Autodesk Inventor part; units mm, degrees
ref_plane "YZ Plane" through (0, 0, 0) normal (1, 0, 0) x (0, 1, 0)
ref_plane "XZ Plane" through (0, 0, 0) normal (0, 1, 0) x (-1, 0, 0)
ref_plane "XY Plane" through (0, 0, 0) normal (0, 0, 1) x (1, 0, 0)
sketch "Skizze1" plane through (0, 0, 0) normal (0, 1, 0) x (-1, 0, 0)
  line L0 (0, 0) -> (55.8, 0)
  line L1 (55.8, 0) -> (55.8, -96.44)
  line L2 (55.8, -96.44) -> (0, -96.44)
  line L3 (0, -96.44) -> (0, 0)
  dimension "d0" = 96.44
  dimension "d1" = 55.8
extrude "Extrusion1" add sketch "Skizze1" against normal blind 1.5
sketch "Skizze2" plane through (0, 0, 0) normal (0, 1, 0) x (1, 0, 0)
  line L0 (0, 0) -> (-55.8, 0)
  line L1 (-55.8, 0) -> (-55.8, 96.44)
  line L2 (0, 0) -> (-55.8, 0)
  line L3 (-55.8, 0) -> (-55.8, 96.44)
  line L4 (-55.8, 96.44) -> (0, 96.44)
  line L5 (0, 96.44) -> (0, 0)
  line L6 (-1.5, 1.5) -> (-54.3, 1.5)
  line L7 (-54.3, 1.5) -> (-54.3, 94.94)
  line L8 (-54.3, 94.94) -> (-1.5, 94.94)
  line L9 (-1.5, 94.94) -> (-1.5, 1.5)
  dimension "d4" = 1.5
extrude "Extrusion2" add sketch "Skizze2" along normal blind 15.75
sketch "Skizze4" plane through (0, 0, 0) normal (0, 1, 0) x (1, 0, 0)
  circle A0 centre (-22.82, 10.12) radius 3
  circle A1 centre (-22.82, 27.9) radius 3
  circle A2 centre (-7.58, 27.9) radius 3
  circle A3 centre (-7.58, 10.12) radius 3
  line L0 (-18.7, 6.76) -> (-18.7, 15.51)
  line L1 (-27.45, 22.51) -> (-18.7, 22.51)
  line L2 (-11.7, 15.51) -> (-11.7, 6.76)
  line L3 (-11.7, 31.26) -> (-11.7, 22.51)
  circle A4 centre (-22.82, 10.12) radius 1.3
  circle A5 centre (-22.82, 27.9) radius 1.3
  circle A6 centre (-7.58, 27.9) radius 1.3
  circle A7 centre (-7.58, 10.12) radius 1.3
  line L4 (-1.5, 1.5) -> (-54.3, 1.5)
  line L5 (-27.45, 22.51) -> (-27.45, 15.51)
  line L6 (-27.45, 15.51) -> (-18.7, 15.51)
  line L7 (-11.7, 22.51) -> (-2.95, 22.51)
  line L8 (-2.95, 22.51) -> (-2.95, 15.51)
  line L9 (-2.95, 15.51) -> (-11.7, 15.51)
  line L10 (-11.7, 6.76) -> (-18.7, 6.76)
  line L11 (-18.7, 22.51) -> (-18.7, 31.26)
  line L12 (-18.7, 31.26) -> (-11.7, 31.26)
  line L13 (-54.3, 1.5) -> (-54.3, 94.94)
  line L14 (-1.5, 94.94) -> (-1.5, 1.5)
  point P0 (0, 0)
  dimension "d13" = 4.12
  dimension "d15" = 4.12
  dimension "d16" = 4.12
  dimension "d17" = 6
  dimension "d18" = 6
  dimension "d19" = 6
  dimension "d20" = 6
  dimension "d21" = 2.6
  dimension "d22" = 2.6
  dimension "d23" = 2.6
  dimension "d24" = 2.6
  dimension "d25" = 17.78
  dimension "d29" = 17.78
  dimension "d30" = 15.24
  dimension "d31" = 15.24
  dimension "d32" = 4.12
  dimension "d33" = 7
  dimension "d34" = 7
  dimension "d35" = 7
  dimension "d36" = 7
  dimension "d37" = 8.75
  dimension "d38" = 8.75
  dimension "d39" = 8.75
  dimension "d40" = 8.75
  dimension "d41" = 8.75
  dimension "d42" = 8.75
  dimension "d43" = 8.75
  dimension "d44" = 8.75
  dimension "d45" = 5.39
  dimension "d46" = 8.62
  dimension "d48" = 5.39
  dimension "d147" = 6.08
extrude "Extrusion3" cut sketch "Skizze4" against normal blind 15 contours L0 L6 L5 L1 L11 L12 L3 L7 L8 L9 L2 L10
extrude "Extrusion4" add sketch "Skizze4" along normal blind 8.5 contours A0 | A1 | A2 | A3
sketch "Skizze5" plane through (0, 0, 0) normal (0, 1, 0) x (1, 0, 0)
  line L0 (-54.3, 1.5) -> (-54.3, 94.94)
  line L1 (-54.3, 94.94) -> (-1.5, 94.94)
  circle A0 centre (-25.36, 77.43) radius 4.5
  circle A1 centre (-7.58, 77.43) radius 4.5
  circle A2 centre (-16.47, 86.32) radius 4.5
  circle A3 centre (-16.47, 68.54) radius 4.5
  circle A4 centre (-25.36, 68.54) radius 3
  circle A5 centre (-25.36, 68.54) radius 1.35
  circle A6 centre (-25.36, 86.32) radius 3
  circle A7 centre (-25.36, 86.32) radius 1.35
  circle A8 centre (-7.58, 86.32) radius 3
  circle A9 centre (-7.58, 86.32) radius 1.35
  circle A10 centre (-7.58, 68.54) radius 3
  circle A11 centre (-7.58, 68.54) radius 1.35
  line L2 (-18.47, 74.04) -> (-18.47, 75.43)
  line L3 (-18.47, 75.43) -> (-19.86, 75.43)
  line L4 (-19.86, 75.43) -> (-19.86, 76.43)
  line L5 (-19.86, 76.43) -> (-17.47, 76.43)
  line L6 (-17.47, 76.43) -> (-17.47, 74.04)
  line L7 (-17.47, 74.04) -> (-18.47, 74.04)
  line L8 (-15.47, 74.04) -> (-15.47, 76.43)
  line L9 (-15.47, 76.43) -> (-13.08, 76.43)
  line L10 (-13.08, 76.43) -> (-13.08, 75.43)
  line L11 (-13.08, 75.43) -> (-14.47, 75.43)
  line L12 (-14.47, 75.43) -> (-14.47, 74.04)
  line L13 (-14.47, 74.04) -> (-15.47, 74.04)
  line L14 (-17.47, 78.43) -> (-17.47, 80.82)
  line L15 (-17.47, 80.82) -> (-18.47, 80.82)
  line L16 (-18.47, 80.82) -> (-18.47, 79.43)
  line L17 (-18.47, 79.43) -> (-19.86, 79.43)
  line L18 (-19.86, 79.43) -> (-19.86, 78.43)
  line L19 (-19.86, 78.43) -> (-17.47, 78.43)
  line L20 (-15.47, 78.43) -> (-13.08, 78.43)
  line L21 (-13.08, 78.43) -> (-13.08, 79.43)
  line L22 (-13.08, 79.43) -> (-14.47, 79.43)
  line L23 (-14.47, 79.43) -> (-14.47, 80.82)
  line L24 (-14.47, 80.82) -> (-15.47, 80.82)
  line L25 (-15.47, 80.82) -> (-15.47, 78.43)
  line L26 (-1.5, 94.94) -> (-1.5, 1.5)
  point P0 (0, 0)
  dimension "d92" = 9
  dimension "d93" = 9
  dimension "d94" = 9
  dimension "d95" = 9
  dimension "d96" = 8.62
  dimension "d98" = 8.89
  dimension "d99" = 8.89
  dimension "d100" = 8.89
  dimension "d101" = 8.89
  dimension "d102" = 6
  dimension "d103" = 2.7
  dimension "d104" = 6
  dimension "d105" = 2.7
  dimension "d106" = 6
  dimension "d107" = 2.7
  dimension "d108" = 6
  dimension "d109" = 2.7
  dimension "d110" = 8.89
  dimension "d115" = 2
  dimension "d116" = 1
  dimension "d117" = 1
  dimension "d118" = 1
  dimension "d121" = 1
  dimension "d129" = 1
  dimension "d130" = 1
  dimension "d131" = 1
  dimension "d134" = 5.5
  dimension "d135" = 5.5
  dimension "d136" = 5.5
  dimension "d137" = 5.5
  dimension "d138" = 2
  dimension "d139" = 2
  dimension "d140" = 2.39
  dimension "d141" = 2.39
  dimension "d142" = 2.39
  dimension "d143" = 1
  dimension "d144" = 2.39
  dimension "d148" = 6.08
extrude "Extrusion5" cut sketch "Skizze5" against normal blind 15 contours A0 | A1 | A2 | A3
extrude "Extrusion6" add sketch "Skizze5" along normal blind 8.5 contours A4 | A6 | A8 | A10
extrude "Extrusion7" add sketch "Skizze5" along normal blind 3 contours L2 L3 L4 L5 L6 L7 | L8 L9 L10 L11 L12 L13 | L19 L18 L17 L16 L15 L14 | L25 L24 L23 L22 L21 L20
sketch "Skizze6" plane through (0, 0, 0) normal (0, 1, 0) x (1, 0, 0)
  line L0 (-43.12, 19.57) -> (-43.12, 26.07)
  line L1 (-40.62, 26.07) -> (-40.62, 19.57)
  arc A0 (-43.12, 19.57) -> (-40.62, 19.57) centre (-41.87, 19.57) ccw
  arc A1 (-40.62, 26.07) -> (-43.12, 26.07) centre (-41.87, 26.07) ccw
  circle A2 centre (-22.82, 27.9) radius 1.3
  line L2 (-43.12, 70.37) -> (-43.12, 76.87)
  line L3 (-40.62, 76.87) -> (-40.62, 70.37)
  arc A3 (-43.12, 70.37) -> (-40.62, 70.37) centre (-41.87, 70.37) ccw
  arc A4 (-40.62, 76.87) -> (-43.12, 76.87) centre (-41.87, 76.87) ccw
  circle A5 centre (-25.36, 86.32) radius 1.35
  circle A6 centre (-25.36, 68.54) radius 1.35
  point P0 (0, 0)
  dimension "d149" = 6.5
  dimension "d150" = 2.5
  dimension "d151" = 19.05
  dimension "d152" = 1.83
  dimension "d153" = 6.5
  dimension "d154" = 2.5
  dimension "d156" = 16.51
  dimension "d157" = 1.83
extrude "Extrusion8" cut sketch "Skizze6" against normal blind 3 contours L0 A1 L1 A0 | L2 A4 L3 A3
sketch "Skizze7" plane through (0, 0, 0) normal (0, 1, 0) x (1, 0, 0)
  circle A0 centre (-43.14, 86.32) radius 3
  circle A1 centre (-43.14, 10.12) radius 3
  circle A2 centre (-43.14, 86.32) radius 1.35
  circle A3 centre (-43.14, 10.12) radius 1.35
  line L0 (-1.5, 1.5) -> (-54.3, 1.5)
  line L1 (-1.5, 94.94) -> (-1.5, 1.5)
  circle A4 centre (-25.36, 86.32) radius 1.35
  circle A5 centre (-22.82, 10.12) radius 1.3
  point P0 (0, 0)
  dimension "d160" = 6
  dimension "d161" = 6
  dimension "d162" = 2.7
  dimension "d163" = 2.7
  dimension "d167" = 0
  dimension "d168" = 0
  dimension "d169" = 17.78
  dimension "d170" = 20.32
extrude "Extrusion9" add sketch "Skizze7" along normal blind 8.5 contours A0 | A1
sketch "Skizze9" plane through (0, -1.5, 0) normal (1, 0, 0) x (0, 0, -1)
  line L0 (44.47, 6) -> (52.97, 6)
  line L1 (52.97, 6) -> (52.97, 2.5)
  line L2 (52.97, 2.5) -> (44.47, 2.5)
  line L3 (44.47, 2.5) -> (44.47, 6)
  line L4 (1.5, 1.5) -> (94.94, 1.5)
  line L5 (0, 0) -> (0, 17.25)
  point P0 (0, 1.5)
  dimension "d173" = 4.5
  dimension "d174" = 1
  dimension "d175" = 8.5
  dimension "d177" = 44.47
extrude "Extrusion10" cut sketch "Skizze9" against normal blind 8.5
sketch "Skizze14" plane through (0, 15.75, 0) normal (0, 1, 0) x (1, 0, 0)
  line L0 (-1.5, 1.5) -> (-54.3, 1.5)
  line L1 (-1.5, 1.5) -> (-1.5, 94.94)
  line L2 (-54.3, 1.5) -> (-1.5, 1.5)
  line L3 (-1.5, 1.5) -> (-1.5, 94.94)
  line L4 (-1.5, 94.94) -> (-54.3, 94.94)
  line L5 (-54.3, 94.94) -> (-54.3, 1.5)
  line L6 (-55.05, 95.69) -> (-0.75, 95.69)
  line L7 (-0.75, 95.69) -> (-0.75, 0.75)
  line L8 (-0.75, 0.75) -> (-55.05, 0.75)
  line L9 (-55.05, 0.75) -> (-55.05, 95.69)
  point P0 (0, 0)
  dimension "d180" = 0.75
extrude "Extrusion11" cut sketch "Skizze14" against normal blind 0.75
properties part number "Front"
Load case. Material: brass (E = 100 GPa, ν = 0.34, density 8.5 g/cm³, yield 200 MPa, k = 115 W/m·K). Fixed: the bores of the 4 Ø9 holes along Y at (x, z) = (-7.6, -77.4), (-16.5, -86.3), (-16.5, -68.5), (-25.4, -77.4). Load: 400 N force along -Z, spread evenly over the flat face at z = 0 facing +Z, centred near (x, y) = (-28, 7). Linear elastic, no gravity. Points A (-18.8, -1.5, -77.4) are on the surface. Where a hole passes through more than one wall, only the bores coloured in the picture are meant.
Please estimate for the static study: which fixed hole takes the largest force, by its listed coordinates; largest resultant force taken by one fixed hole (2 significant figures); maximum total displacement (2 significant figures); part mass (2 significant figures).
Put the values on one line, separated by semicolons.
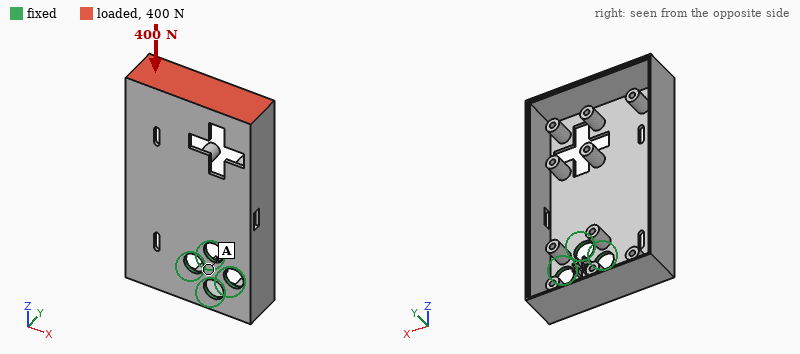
(-25.4, -77.4); 270 N; 0.48 mm; 140 g
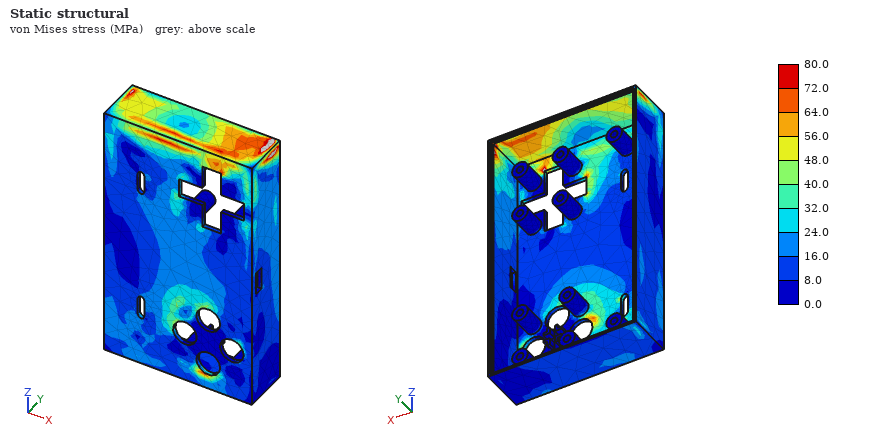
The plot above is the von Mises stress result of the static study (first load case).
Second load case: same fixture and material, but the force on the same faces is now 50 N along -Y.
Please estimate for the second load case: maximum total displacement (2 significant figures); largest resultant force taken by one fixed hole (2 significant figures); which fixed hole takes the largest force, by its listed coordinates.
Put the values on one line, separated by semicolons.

0.66 mm; 120 N; (-16.5, -86.3)
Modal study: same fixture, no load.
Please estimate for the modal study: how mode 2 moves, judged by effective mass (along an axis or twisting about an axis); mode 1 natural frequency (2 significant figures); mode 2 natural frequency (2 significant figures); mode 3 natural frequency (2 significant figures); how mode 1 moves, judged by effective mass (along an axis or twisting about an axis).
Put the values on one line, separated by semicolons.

along Y; 240 Hz; 630 Hz; 1200 Hz; along Y
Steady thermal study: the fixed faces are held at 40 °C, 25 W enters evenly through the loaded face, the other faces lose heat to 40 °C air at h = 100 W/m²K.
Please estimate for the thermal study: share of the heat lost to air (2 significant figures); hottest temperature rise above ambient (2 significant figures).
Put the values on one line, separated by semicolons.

92 %; 55 K
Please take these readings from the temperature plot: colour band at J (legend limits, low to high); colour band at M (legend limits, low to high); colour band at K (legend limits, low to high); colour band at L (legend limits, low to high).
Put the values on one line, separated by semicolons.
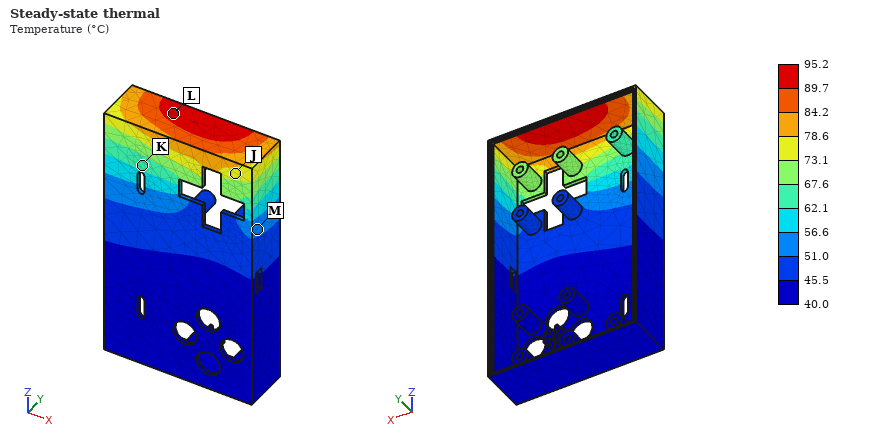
73.1 to 78.6 °C; 51.0 to 56.6 °C; 62.1 to 67.6 °C; 89.7 to 95.2 °C
